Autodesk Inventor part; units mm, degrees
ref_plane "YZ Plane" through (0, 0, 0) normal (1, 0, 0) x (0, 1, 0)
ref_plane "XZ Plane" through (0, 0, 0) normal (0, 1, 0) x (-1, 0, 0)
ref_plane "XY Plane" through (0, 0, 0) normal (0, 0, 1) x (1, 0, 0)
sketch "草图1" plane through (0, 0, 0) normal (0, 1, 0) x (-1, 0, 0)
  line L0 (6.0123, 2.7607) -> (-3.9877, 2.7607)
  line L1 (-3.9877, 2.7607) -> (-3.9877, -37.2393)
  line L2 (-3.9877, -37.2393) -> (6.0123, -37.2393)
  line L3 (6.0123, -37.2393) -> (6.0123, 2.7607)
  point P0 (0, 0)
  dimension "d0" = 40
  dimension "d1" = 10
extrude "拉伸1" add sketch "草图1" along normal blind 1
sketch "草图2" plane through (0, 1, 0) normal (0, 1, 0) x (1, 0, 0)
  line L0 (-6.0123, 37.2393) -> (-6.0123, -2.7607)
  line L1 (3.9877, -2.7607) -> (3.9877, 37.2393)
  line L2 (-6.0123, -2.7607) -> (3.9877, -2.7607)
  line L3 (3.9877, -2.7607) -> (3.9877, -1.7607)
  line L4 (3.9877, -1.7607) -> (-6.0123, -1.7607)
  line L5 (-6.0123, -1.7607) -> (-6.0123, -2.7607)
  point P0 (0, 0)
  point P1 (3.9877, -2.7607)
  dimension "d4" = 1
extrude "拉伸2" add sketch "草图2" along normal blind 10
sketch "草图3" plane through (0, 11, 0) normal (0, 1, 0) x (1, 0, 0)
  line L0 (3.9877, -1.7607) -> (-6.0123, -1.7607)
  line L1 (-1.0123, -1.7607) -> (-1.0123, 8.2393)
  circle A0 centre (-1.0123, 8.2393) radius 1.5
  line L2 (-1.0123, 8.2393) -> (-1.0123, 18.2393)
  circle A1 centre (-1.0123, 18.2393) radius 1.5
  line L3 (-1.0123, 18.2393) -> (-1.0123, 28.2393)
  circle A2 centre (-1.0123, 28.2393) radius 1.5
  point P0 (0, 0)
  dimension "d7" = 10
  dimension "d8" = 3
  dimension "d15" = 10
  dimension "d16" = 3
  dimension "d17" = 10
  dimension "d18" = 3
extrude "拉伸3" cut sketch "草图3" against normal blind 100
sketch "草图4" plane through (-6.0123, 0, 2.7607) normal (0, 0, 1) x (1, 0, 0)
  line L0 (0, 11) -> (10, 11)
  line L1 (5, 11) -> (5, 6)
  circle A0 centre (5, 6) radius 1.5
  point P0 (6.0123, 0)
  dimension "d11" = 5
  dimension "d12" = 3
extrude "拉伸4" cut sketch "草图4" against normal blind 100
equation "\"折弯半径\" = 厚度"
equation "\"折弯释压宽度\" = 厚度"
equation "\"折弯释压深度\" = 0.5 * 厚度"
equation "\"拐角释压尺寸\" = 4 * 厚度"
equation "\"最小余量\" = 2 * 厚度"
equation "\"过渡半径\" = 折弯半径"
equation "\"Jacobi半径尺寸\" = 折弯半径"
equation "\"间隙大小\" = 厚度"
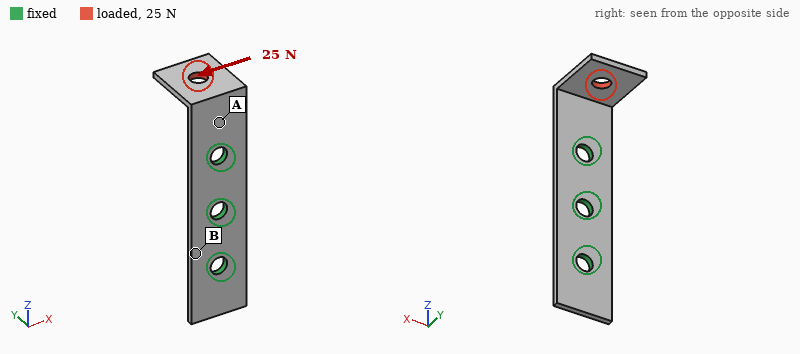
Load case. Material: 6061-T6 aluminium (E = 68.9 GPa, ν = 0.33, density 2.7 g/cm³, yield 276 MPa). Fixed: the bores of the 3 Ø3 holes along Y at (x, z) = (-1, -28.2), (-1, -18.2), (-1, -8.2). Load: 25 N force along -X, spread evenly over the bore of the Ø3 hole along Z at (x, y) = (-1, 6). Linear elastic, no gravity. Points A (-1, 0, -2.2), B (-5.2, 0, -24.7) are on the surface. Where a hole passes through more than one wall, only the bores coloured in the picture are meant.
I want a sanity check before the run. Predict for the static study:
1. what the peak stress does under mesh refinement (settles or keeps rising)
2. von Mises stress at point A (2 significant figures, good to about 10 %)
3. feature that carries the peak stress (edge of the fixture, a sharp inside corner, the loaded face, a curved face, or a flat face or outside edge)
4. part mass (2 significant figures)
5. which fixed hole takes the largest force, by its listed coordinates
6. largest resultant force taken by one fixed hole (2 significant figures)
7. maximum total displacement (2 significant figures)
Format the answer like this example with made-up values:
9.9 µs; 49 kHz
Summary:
keeps rising; 60 MPa; edge of the fixture; 1.3 g; (-1, -8.2); 37 N; 0.15 mm
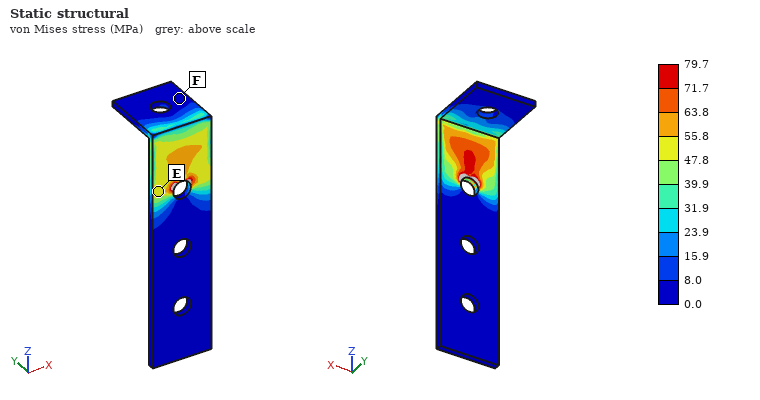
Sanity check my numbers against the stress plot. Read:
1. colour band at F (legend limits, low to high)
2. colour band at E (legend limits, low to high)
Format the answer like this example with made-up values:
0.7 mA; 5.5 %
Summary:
0.0 to 8.0 MPa; 47.8 to 55.8 MPa
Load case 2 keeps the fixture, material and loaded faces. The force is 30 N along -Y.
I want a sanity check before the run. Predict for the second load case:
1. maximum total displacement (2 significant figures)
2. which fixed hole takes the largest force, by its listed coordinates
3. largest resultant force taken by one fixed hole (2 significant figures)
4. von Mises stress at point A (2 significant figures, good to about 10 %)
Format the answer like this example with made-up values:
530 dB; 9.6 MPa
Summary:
0.29 mm; (-1, -8.2); 32 N; 69 MPa
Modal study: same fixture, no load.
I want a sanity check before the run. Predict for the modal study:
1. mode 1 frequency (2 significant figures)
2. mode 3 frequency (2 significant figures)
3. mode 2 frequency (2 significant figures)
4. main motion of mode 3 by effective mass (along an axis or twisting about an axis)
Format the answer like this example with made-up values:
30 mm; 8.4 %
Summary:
2800 Hz; 7600 Hz; 4500 Hz; along Y
